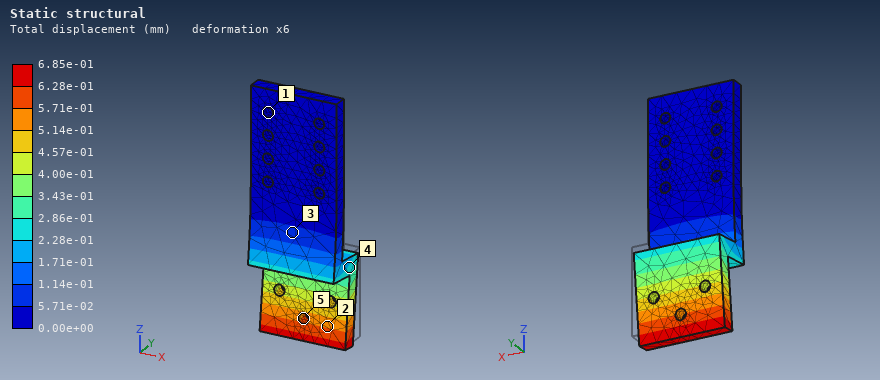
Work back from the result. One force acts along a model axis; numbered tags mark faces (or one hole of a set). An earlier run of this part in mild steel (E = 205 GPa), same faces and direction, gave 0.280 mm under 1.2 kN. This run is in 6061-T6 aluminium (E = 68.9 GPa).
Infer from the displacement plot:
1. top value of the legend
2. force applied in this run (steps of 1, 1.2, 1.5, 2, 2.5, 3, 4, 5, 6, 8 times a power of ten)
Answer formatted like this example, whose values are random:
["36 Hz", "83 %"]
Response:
["6.85e-01 mm", "1 kN"]
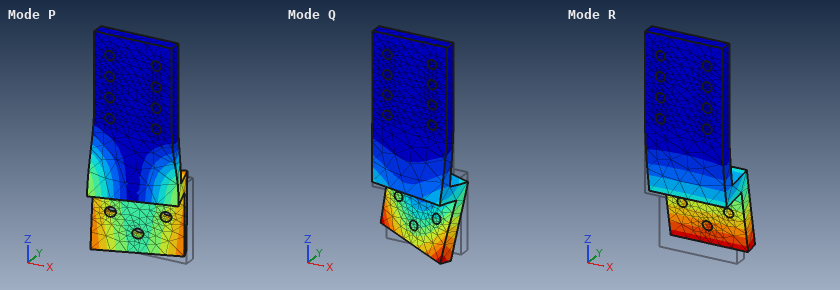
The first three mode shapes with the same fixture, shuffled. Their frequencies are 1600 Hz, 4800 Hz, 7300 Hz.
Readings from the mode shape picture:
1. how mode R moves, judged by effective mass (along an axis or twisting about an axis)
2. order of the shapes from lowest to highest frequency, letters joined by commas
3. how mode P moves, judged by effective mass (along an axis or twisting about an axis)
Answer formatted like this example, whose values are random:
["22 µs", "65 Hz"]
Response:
["along Y", "R, P, Q", "along X"]
